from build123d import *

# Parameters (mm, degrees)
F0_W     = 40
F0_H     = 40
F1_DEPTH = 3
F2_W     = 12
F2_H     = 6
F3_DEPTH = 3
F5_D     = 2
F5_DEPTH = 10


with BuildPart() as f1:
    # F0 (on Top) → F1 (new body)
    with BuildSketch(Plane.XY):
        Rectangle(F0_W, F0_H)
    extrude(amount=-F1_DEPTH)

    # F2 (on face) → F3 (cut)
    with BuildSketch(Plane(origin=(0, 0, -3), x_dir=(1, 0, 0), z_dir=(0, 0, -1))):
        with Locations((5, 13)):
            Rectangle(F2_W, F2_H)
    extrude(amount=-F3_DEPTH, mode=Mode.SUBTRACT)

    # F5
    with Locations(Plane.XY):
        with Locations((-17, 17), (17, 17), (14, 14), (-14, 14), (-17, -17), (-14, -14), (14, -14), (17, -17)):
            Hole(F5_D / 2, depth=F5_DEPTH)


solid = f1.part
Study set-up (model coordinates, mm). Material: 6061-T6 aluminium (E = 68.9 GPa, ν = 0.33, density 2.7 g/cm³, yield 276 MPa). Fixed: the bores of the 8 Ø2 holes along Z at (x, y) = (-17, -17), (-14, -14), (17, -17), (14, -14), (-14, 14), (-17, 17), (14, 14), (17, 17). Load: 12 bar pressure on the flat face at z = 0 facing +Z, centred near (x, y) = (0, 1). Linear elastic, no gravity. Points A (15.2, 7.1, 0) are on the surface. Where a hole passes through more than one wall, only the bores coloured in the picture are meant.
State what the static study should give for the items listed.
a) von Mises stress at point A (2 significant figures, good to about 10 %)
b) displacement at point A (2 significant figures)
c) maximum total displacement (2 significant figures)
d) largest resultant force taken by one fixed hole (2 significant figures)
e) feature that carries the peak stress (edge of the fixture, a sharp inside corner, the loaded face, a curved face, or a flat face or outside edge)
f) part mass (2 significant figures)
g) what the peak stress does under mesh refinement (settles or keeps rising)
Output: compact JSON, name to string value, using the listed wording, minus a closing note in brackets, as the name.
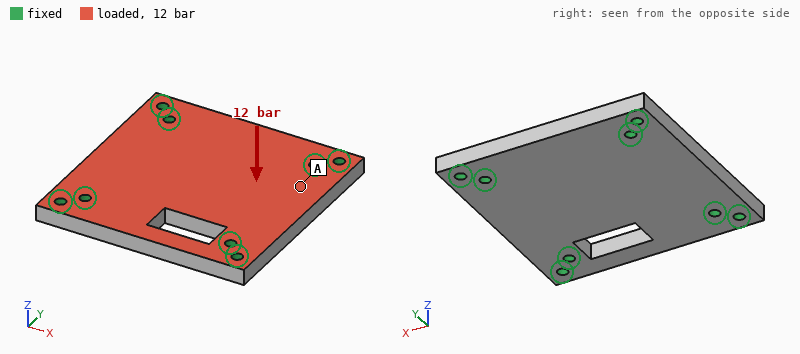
{"von Mises stress at point A": "17 MPa", "displacement at point A": "12 µm", "maximum total displacement": "34 µm", "largest resultant force taken by one fixed hole": "510 N", "feature that carries the peak stress": "edge of the fixture", "part mass": "12 g", "what the peak stress does under mesh refinement": "keeps rising"}
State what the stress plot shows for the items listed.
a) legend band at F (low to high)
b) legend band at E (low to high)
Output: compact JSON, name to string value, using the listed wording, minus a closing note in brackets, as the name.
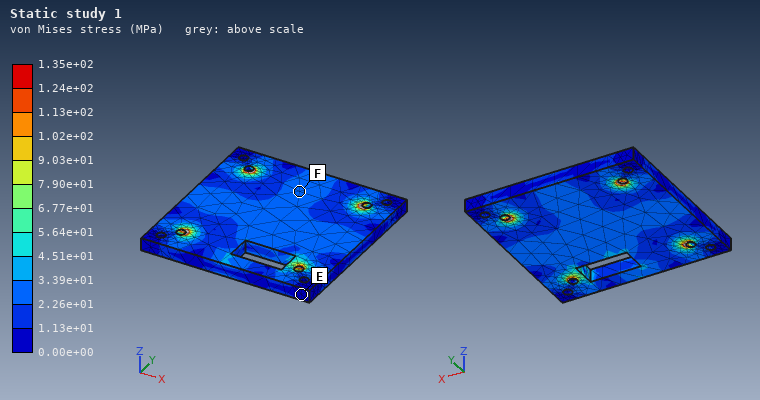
{"legend band at F": "2.26e+01 to 3.39e+01 MPa", "legend band at E": "0.00e+00 to 1.13e+01 MPa"}
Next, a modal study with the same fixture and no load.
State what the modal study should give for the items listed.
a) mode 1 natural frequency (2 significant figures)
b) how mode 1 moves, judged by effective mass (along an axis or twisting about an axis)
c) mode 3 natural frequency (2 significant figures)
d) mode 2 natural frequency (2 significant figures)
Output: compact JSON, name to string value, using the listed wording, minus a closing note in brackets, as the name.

{"mode 1 natural frequency": "13 kHz", "how mode 1 moves, judged by effective mass": "along Z", "mode 3 natural frequency": "19 kHz", "mode 2 natural frequency": "19 kHz"}
